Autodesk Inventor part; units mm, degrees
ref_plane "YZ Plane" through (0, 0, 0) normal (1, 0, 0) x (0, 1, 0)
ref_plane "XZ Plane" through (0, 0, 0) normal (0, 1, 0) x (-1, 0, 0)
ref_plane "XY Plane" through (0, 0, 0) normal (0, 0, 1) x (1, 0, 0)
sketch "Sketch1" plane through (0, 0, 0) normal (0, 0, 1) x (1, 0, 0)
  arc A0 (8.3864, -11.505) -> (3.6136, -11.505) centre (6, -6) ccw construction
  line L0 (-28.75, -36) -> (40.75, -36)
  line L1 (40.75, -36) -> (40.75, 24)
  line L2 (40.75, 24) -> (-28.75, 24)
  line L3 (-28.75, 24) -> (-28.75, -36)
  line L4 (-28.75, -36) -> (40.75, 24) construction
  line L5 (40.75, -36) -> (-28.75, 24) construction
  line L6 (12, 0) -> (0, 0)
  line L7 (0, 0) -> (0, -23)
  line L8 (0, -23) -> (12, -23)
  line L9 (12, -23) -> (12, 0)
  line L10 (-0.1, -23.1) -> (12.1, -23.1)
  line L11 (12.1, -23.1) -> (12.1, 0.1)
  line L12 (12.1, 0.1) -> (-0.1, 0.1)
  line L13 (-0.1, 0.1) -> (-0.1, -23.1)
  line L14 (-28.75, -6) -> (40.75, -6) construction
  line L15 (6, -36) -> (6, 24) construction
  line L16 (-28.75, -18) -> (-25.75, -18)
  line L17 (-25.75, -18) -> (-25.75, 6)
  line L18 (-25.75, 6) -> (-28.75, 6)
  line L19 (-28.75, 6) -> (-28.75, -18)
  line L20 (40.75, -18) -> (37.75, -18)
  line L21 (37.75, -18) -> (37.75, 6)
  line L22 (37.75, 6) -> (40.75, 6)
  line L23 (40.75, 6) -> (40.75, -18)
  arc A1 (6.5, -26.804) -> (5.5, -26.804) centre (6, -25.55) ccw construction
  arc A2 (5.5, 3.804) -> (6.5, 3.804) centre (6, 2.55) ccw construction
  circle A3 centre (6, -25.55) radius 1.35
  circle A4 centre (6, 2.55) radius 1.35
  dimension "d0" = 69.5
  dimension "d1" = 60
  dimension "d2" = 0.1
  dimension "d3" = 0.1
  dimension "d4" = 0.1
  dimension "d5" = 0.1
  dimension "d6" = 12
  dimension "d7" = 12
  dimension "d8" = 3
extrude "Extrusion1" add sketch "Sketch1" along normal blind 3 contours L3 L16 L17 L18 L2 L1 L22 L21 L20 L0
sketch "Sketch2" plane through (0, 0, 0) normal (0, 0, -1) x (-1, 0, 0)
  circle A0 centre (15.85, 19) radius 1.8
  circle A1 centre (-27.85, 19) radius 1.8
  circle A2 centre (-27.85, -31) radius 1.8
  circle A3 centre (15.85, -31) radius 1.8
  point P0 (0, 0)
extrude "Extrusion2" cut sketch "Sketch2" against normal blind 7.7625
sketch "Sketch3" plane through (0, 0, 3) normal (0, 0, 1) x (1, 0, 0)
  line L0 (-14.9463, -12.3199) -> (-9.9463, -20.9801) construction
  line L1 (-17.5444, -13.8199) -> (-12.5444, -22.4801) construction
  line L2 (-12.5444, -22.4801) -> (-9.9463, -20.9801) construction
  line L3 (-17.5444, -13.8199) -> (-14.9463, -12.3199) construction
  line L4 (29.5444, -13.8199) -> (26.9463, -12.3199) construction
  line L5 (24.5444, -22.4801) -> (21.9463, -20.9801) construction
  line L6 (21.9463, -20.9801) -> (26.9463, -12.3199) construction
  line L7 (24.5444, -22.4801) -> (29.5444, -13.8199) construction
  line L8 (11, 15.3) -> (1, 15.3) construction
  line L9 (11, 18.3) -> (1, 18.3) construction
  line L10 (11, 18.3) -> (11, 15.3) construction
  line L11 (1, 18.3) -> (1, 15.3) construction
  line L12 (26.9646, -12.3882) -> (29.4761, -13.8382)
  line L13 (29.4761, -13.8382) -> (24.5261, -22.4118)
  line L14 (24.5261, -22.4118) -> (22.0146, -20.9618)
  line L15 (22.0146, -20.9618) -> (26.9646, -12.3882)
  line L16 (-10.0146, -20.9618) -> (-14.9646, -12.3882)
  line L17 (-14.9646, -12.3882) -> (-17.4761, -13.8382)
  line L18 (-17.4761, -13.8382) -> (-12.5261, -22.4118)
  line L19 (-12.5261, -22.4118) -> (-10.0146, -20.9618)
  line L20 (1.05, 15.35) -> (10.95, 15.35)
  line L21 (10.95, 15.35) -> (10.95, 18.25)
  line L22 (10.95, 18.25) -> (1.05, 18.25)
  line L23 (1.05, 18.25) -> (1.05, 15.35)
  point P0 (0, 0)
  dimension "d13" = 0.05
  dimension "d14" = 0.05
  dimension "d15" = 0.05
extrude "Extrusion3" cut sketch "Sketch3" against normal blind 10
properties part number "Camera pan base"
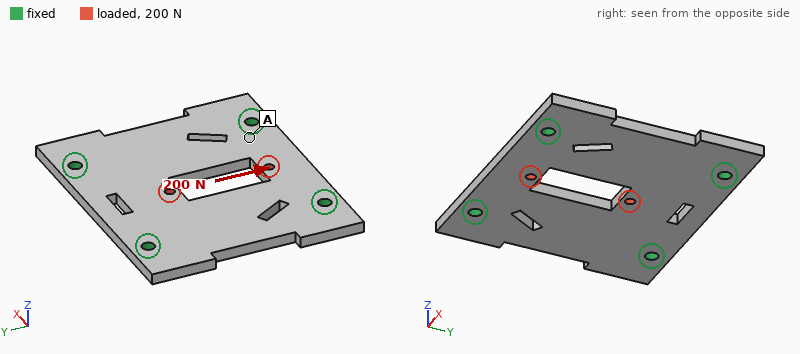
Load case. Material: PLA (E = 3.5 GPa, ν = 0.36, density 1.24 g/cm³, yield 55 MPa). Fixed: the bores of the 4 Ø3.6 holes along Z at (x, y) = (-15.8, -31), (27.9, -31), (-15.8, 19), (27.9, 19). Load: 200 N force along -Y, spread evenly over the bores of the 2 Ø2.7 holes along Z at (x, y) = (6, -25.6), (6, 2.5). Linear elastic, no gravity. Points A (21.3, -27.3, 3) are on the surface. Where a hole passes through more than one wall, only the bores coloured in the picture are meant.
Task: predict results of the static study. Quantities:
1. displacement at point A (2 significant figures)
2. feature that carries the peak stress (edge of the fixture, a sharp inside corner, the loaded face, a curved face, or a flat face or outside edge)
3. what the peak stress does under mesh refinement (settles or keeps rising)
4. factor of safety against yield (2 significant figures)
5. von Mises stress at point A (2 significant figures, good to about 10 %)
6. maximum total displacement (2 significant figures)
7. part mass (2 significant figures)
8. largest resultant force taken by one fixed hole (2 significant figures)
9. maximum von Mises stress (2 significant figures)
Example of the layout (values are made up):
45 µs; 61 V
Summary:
6.3 µm; a flat face or outside edge; settles; 4.1; 1.3 MPa; 34 µm; 13 g; 62 N; 13 MPa
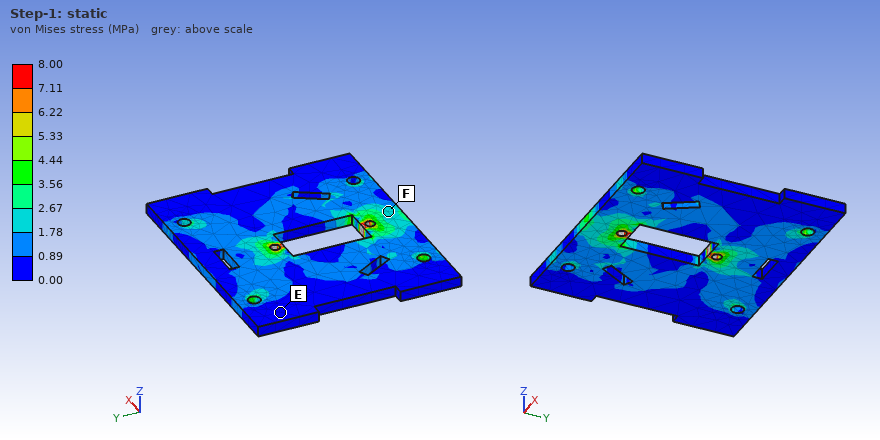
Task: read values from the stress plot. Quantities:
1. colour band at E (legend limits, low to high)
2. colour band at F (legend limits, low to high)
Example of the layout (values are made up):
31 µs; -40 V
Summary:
0.00 to 0.89 MPa; 1.78 to 2.67 MPa
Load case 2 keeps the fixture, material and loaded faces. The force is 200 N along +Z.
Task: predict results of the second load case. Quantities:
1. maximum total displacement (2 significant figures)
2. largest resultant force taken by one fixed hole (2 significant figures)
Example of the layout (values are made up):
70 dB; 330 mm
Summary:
0.76 mm; 61 N
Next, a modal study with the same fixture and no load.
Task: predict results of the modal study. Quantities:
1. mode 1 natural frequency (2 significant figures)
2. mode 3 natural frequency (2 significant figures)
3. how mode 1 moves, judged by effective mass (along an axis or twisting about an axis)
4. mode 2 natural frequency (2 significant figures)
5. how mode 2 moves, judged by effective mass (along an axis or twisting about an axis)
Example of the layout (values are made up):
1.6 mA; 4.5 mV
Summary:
1700 Hz; 2300 Hz; along Z; 2100 Hz; twisting about Y
